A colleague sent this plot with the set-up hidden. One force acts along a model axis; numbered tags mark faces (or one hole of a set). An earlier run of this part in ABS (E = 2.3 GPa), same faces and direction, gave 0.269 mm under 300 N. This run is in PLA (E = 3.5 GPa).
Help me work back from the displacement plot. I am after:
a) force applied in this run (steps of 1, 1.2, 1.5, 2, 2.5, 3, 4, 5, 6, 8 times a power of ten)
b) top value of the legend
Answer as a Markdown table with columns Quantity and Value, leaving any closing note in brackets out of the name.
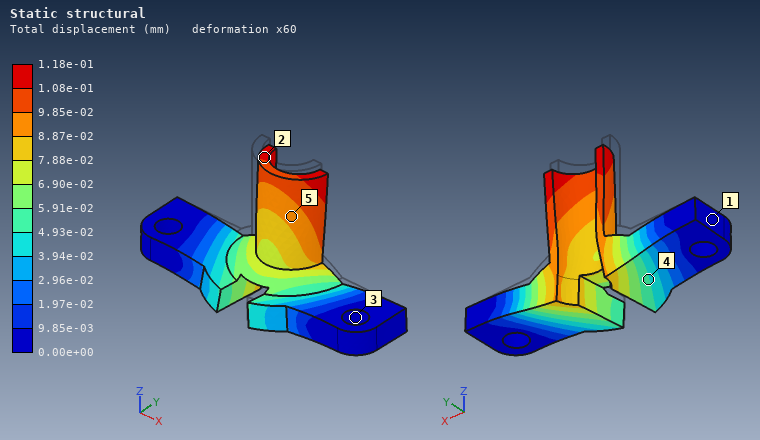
| Quantity | Value |
|---|---|
| force applied in this run | 200 N |
| top value of the legend | 1.18e-01 mm |
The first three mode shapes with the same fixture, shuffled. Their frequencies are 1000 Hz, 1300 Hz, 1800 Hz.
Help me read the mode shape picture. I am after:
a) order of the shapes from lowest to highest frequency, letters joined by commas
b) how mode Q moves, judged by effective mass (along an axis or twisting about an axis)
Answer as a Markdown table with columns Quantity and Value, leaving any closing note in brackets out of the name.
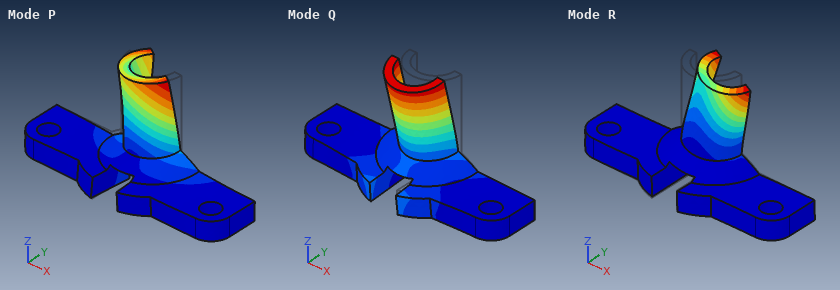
| Quantity | Value |
|---|---|
| order of the shapes from lowest to highest frequency, letters joined by commas | Q, R, P |
| how mode Q moves, judged by effective mass | along Y |
